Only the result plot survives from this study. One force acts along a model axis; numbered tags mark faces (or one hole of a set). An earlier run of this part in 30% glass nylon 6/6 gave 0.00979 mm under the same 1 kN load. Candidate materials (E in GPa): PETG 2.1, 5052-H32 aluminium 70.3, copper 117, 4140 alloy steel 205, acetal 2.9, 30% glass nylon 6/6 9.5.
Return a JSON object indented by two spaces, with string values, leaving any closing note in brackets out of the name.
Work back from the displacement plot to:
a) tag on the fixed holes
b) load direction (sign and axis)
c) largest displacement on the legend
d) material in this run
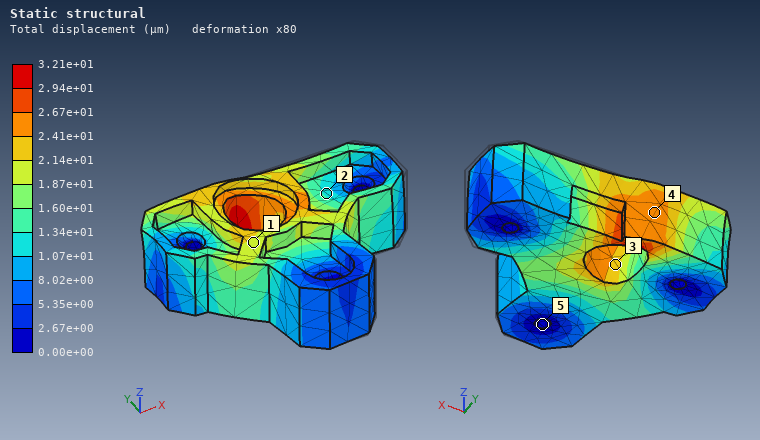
{
  "tag on the fixed holes": "5",
  "load direction": "-X",
  "largest displacement on the legend": "3.21e+01 µm",
  "material in this run": "acetal"
}
